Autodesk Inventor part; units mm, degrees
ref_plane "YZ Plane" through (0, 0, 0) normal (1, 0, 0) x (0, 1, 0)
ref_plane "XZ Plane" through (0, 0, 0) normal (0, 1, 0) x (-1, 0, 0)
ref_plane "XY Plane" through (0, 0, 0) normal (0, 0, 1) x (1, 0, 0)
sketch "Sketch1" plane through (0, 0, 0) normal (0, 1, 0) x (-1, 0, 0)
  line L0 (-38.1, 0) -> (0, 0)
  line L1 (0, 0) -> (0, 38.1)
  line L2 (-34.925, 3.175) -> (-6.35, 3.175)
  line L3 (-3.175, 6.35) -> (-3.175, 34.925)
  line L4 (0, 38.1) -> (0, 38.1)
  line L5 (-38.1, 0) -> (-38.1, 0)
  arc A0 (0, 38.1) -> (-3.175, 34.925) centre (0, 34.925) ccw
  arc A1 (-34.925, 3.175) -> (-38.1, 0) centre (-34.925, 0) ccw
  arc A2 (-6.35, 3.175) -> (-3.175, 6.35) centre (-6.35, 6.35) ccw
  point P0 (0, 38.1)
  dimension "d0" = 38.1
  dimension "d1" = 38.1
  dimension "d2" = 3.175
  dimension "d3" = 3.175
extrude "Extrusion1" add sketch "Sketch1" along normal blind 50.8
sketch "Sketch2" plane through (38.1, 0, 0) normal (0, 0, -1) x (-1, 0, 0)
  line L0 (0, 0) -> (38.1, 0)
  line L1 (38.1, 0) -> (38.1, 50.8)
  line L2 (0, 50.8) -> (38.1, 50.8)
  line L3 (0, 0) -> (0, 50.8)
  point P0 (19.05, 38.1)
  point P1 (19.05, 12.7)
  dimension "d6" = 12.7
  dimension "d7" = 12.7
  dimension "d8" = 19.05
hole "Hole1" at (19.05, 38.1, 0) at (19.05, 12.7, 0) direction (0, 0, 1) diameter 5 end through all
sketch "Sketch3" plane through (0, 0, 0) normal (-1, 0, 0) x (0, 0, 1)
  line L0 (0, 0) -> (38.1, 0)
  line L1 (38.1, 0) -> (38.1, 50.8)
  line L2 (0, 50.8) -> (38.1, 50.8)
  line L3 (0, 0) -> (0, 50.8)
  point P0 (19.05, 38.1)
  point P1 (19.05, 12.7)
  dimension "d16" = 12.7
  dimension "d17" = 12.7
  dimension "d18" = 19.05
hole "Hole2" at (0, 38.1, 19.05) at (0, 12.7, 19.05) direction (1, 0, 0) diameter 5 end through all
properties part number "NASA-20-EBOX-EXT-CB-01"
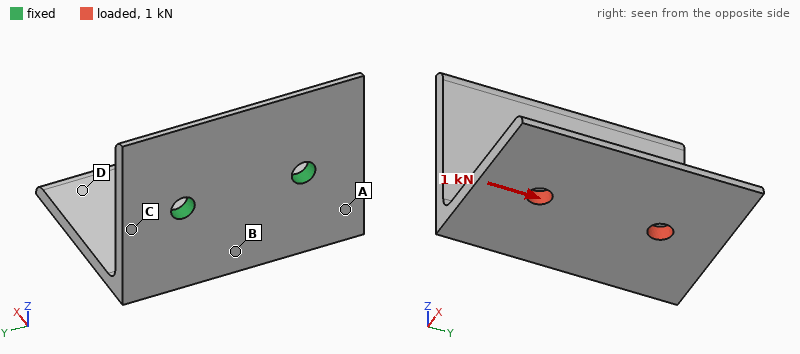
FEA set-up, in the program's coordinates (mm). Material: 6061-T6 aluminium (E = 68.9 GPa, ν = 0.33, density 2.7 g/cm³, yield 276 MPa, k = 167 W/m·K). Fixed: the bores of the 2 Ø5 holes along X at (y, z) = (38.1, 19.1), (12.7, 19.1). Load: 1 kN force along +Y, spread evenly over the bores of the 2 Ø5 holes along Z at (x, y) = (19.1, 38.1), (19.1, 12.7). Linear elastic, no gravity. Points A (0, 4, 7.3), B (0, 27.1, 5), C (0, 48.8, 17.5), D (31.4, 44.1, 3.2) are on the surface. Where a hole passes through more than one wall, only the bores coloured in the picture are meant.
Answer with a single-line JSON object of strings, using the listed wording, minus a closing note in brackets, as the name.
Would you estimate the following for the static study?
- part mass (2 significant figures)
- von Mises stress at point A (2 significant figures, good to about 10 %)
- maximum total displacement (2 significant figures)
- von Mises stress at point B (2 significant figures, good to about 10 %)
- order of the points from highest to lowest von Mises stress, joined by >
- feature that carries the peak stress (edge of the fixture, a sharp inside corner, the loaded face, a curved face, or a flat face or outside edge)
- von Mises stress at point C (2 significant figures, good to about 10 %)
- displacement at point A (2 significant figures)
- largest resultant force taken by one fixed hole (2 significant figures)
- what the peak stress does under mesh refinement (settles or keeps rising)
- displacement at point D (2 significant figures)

{"part mass": "31 g", "von Mises stress at point A": "28 MPa", "maximum total displacement": "0.29 mm", "von Mises stress at point B": "50 MPa", "order of the points from highest to lowest von Mises stress, joined by >": "C > B > A > D", "feature that carries the peak stress": "edge of the fixture", "von Mises stress at point C": "71 MPa", "displacement at point A": "0.084 mm", "largest resultant force taken by one fixed hole": "950 N", "what the peak stress does under mesh refinement": "keeps rising", "displacement at point D": "0.23 mm"}
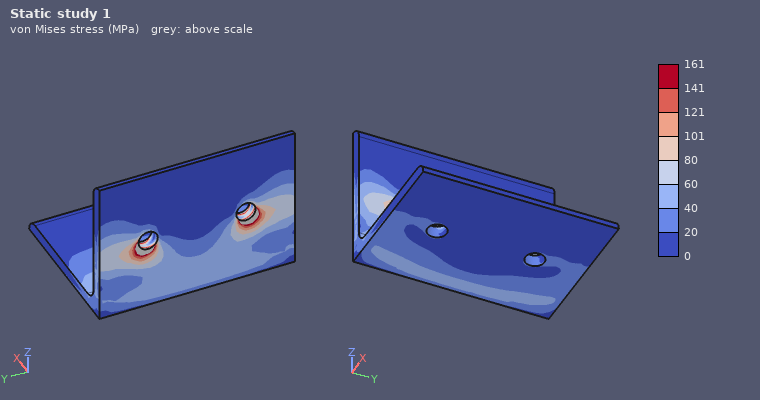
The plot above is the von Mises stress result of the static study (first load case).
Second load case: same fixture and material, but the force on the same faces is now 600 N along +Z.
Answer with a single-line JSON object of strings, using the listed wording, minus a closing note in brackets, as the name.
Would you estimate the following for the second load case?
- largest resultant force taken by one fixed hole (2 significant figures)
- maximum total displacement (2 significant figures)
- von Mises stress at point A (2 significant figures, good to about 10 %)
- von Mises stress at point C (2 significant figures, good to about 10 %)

{"largest resultant force taken by one fixed hole": "310 N", "maximum total displacement": "0.81 mm", "von Mises stress at point A": "110 MPa", "von Mises stress at point C": "66 MPa"}
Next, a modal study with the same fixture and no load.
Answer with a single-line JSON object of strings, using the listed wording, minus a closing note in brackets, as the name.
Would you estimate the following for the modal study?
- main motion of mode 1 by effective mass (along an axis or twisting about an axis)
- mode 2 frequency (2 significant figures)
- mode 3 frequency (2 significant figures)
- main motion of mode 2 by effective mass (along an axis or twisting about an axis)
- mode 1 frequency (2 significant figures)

{"main motion of mode 1 by effective mass": "along Z", "mode 2 frequency": "2400 Hz", "mode 3 frequency": "3900 Hz", "main motion of mode 2 by effective mass": "along Y", "mode 1 frequency": "1200 Hz"}
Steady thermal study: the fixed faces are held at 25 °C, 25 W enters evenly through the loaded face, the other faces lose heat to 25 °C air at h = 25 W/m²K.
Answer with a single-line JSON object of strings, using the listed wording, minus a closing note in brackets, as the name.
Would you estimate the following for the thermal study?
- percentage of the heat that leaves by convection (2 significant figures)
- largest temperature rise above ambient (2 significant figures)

{"percentage of the heat that leaves by convection": "12 %", "largest temperature rise above ambient": "32 K"}
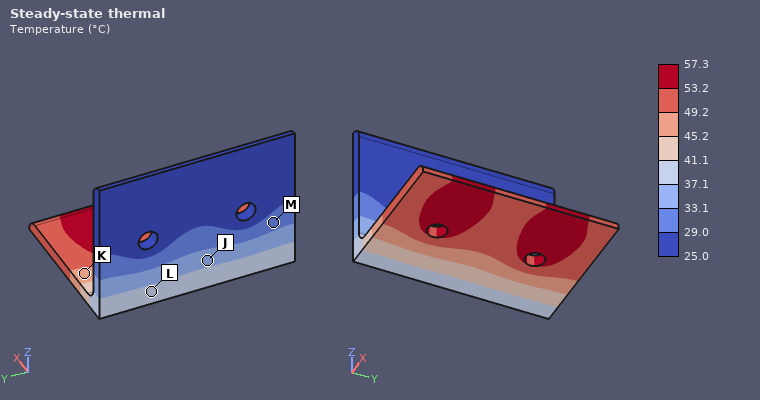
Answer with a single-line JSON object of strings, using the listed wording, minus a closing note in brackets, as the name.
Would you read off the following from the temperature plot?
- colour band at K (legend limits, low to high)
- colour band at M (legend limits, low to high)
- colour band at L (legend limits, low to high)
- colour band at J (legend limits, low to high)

{"colour band at K": "45.2 to 49.2 °C", "colour band at M": "29.0 to 33.1 °C", "colour band at L": "37.1 to 41.1 °C", "colour band at J": "33.1 to 37.1 °C"}
